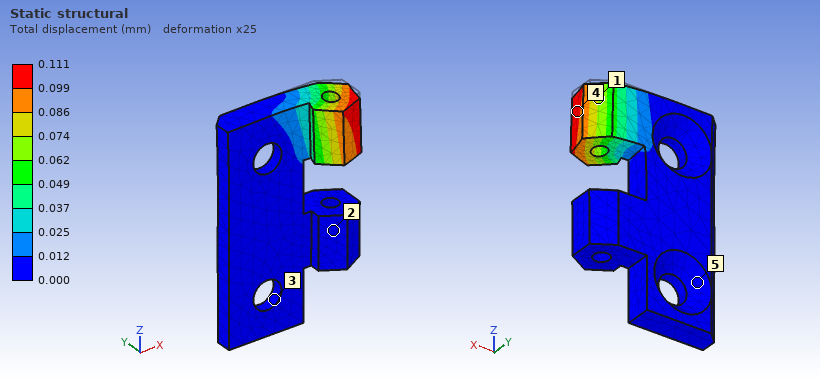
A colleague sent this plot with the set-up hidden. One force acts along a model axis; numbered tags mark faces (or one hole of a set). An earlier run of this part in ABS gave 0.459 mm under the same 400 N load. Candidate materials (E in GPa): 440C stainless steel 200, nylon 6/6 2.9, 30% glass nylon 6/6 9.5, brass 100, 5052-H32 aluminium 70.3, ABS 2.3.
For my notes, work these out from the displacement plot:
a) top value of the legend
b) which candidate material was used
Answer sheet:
0.111 mm
30% glass nylon 6/6
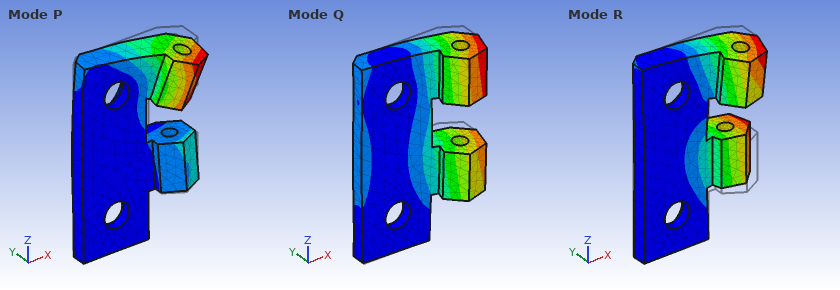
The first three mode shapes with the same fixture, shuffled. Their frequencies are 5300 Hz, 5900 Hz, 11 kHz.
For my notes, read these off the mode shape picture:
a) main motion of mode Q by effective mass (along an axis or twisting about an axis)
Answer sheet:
along Y
